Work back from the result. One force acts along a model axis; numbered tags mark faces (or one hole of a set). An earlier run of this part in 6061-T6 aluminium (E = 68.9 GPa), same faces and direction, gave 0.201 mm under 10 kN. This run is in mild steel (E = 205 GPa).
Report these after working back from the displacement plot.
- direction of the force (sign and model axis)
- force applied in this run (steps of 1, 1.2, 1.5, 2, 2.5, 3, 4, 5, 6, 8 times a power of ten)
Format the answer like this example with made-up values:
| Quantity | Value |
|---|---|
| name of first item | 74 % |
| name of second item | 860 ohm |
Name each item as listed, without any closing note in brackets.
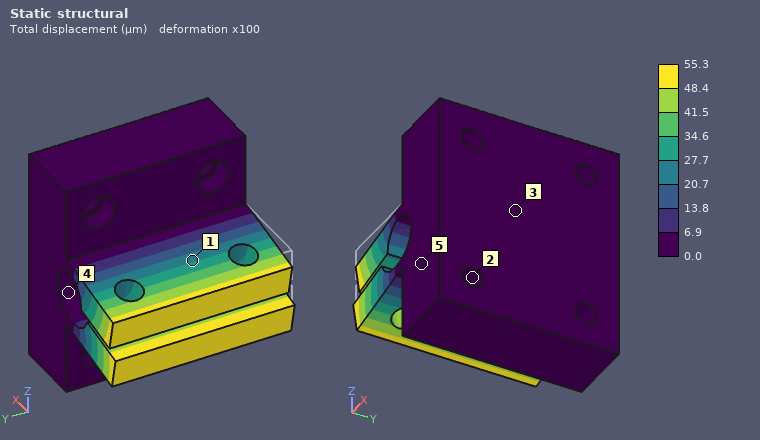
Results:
| Quantity | Value |
|---|---|
| direction of the force | -Z |
| force applied in this run | 8 kN |
